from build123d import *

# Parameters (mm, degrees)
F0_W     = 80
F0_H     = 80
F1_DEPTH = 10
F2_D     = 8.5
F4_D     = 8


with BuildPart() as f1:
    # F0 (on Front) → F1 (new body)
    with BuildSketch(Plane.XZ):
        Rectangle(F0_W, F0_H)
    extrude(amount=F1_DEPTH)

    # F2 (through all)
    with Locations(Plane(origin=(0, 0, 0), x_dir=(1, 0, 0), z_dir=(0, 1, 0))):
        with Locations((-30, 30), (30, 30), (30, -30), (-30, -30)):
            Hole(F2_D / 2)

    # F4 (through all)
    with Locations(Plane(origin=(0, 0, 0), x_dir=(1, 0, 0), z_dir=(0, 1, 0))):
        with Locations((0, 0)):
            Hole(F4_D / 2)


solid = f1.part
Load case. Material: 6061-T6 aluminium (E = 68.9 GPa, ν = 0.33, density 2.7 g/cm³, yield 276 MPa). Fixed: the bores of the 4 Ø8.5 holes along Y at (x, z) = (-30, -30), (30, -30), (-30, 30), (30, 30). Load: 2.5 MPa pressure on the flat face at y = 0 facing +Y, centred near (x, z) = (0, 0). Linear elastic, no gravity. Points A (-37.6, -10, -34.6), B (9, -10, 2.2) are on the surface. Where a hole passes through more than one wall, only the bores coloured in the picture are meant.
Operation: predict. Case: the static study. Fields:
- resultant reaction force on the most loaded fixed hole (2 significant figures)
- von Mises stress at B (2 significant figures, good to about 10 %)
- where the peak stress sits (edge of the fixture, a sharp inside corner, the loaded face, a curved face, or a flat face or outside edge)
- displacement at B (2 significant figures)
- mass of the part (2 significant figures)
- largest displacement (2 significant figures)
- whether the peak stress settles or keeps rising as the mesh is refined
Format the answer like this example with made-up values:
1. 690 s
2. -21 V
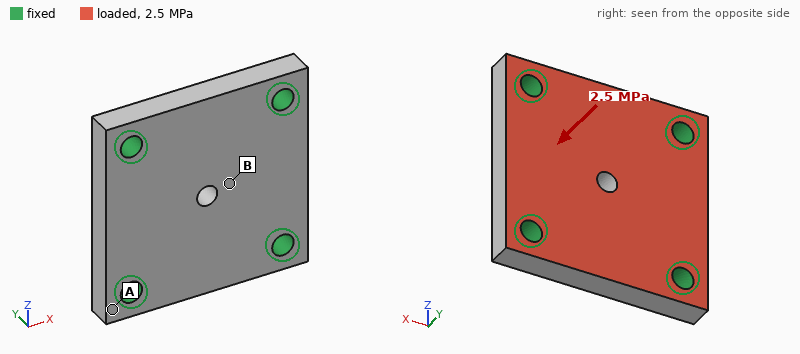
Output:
1. 3.8 kN
2. 25 MPa
3. edge of the fixture
4. 35 µm
5. 170 g
6. 38 µm
7. keeps rising
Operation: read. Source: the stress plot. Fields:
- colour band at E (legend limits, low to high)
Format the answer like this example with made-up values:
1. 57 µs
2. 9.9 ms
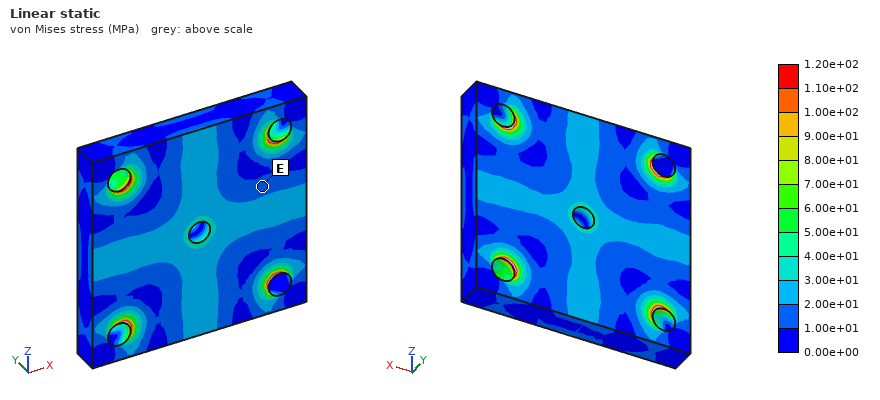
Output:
1. 1.00e+01 to 2.00e+01 MPa
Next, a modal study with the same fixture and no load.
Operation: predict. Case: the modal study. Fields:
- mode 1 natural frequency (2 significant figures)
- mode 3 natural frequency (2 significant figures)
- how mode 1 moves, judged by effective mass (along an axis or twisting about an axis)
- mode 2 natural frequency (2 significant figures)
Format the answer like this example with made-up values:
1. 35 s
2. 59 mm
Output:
1. 9700 Hz
2. 15 kHz
3. along Y
4. 15 kHz
